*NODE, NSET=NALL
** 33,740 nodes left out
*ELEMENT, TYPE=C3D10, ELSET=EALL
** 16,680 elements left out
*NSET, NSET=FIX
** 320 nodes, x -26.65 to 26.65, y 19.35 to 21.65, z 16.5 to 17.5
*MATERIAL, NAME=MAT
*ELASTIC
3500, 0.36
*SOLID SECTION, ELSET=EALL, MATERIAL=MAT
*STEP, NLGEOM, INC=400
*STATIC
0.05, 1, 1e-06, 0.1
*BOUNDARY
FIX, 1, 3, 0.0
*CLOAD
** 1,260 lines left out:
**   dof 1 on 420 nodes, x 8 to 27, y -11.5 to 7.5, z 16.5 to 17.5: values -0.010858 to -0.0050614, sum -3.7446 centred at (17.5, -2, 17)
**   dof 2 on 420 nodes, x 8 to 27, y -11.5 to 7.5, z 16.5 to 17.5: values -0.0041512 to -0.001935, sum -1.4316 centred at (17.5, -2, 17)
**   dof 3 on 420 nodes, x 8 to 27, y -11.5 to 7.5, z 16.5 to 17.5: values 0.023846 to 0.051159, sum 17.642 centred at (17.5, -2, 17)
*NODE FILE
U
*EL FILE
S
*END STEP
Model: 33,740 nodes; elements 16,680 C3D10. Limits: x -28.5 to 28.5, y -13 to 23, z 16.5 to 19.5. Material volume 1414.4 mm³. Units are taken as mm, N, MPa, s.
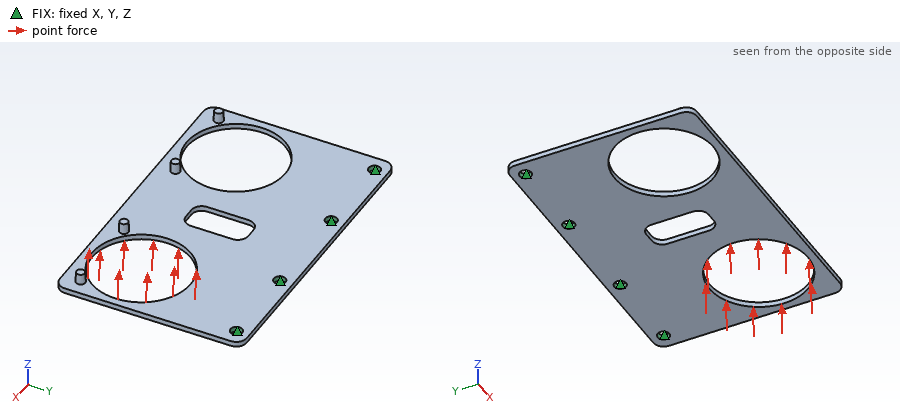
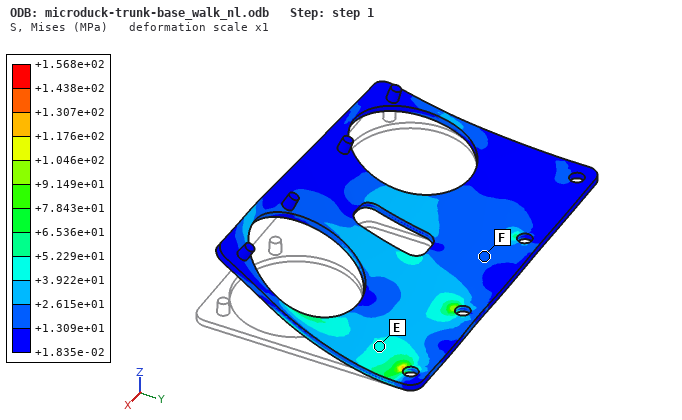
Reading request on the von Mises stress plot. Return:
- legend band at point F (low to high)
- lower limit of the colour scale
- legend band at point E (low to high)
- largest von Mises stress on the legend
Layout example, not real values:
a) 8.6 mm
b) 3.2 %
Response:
a) +1.309e+01 to +2.615e+01 MPa
b) +1.835e-02 MPa
c) +3.922e+01 to +5.229e+01 MPa
d) +1.568e+02 MPa
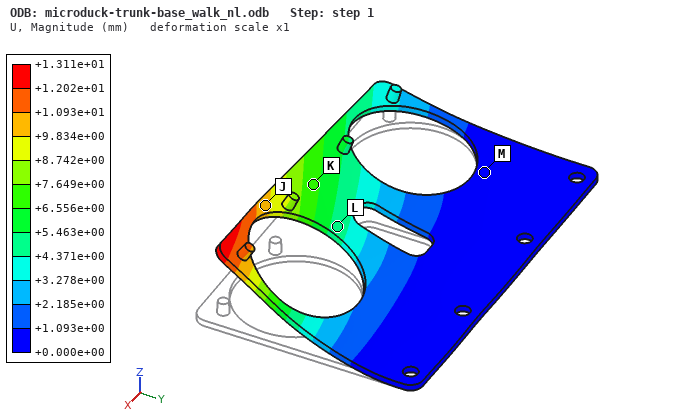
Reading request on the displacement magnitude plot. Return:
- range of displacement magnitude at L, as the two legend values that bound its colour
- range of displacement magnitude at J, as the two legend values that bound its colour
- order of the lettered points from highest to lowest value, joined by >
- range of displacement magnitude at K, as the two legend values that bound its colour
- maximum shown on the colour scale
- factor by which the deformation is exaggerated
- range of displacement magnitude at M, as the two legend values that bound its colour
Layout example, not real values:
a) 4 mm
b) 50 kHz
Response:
a) +4.371e+00 to +5.463e+00 mm
b) +9.834e+00 to +1.093e+01 mm
c) J > K > L > M
d) +6.556e+00 to +7.649e+00 mm
e) +1.311e+01 mm
f) 1
g) +0.000e+00 to +1.093e+00 mm
